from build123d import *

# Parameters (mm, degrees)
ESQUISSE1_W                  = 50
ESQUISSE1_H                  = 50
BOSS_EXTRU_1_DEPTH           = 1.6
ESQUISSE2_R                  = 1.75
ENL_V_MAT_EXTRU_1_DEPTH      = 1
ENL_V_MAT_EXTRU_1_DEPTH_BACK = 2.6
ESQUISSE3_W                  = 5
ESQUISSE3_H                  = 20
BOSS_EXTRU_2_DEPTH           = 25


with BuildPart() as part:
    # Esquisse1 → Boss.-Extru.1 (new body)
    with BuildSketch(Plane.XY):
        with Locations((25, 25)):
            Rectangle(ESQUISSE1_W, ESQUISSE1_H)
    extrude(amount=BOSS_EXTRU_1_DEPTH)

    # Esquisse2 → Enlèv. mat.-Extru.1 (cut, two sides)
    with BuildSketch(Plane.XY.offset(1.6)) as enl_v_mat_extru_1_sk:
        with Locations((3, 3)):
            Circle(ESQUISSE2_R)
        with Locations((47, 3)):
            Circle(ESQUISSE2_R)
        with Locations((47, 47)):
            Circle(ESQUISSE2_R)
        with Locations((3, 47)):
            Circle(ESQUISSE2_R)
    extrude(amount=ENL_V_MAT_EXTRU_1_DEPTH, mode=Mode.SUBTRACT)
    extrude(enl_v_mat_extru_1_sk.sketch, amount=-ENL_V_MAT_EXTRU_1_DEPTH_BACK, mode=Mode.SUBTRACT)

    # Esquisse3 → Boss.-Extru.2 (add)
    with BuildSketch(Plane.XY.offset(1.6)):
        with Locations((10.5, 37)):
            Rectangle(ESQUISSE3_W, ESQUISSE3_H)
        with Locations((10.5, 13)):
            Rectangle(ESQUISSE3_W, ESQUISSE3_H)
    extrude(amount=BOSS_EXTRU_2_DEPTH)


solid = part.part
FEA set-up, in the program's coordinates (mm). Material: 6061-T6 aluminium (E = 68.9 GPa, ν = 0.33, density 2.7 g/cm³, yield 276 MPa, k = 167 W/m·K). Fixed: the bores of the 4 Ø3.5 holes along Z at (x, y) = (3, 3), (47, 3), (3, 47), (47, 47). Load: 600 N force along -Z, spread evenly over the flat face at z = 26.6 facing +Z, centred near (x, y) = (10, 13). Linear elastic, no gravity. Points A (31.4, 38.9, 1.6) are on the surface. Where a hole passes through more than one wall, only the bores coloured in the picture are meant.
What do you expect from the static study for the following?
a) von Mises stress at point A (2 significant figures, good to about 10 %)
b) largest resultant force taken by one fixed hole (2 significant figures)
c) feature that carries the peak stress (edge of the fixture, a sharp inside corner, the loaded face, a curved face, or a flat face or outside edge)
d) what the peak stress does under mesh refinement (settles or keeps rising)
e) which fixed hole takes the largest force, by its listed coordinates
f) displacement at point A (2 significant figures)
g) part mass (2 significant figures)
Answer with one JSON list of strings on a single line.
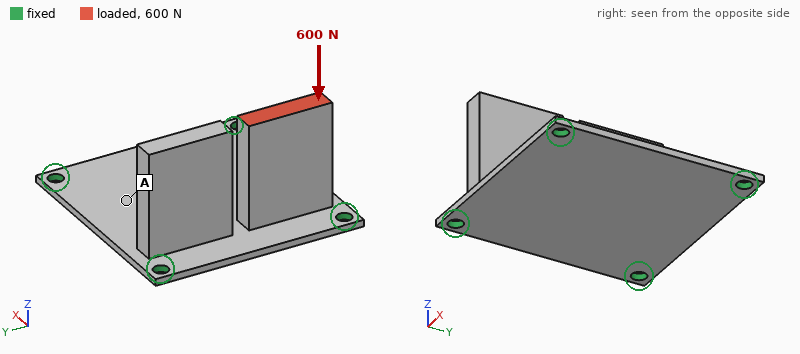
["21 MPa", "430 N", "edge of the fixture", "keeps rising", "(3, 3)", "0.088 mm", "24 g"]
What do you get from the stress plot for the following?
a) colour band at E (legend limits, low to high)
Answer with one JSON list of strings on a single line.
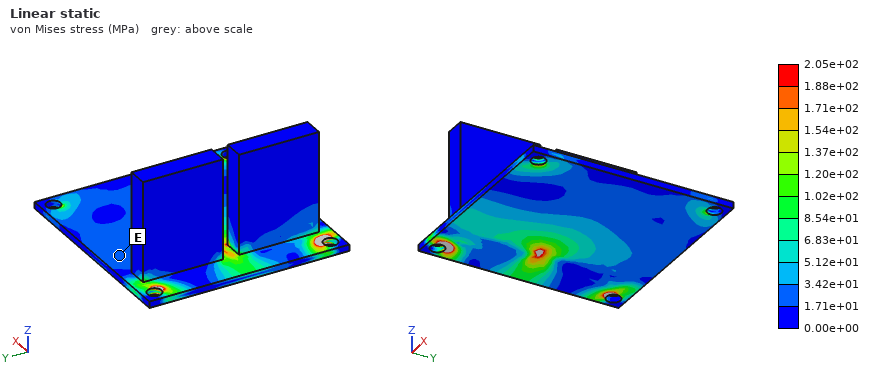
["1.71e+01 to 3.42e+01 MPa"]
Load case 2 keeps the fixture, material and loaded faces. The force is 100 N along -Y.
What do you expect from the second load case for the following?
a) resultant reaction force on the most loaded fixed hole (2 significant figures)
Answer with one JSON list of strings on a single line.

["77 N"]
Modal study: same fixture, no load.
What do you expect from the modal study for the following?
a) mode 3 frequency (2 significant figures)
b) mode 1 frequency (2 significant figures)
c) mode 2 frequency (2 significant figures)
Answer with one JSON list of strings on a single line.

["2300 Hz", "1400 Hz", "1700 Hz"]
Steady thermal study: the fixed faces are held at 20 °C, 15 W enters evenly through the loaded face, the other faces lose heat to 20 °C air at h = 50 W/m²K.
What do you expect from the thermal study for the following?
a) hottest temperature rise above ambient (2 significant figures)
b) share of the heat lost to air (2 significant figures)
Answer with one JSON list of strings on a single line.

["36 K", "23 %"]
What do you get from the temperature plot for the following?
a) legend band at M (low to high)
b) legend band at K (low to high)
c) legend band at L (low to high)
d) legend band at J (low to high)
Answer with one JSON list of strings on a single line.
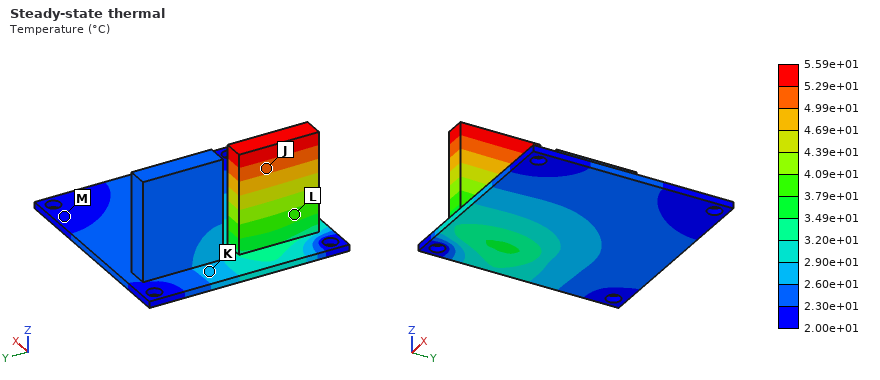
["2.00e+01 to 2.30e+01 °C", "2.60e+01 to 2.90e+01 °C", "3.79e+01 to 4.09e+01 °C", "4.99e+01 to 5.29e+01 °C"]
